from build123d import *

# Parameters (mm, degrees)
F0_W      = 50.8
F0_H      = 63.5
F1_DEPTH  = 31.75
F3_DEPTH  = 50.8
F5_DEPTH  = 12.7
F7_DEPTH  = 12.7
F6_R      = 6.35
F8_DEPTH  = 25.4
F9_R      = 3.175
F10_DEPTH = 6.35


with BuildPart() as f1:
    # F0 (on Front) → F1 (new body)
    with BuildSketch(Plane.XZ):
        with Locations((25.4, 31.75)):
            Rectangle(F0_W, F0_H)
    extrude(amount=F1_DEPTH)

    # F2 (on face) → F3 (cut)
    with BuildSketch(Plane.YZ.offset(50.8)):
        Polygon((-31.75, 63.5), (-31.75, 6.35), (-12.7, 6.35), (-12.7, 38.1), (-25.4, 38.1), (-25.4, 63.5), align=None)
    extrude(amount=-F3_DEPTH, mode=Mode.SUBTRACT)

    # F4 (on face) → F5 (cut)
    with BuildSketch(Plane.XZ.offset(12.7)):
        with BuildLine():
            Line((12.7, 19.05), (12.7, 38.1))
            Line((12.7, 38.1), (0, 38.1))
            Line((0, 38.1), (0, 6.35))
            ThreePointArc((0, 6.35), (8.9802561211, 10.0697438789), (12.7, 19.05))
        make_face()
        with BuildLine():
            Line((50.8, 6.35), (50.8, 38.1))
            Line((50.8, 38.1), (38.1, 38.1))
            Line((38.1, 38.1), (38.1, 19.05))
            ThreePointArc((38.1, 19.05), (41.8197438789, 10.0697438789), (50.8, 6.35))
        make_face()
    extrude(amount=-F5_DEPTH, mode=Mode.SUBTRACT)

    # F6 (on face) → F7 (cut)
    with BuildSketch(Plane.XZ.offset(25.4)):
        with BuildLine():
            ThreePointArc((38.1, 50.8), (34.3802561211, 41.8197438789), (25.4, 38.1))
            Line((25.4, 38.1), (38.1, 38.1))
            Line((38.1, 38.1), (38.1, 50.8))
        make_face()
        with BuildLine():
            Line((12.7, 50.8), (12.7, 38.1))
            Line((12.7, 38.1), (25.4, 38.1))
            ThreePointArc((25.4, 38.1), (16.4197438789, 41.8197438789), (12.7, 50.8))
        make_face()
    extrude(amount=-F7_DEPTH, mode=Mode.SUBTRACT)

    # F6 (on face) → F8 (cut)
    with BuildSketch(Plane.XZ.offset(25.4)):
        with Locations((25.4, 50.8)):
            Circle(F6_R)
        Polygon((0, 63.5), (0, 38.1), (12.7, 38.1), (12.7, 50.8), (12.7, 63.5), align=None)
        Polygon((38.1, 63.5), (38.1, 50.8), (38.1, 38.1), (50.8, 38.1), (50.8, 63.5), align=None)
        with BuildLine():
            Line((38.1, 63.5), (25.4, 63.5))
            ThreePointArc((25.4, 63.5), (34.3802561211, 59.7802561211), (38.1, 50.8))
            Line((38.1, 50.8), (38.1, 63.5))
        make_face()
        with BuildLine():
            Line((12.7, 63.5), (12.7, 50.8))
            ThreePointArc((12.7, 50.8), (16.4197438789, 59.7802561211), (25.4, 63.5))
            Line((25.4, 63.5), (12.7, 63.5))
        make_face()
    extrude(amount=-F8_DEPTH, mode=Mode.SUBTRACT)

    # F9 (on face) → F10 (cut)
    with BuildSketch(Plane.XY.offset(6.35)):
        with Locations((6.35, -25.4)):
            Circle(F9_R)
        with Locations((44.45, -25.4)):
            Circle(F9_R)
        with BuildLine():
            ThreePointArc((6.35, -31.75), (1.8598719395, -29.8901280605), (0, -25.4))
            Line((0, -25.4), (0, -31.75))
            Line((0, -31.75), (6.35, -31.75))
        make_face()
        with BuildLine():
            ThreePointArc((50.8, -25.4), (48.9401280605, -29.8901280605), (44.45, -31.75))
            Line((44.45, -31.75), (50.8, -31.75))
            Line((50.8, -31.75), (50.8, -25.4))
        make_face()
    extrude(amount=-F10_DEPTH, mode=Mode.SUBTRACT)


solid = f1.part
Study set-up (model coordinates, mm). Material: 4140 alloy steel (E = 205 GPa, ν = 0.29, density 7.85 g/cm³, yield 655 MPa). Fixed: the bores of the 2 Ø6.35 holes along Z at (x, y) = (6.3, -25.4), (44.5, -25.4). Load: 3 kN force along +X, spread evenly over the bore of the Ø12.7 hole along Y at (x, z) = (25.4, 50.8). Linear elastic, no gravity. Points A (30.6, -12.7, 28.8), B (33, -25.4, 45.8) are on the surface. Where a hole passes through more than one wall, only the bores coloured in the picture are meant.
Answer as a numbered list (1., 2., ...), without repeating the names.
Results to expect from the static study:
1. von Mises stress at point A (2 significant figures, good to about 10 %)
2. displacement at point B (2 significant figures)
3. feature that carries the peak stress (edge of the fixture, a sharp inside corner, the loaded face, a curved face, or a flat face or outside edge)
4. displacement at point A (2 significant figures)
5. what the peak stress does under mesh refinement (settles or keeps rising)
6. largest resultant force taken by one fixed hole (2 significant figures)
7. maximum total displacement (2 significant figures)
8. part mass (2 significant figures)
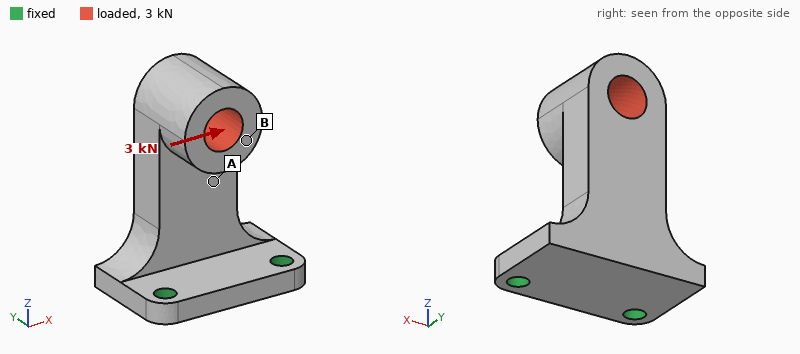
1. 58 MPa
2. 0.12 mm
3. edge of the fixture
4. 0.057 mm
5. keeps rising
6. 4.2 kN
7. 0.16 mm
8. 250 g
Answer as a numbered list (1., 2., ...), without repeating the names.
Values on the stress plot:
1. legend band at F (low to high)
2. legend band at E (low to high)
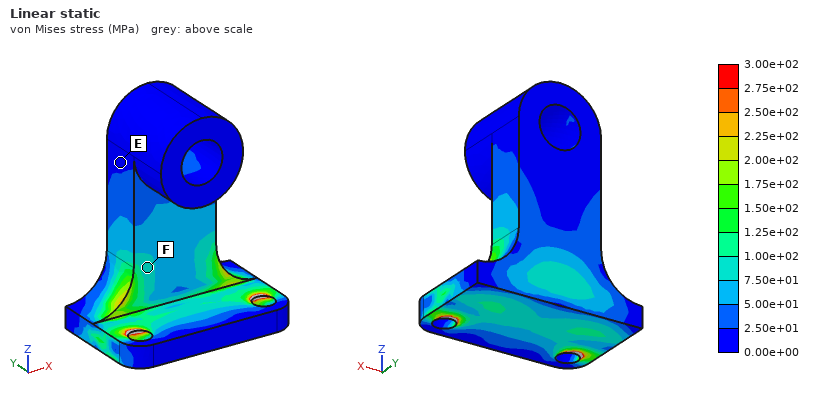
1. 7.50e+01 to 1.00e+02 MPa
2. 0.00e+00 to 2.50e+01 MPa
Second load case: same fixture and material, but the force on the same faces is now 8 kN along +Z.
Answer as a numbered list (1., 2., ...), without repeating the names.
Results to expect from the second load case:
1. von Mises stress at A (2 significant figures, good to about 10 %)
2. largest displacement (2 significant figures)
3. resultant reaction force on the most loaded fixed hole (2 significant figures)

1. 96 MPa
2. 0.11 mm
3. 4.0 kN
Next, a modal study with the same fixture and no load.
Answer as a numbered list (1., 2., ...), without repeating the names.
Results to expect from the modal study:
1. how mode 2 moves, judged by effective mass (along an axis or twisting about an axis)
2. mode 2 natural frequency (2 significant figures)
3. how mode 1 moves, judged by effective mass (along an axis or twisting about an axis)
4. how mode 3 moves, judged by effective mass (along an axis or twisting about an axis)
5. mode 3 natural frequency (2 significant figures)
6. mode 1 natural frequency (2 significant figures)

1. along X
2. 2600 Hz
3. along Y
4. along Z
5. 4900 Hz
6. 1100 Hz
